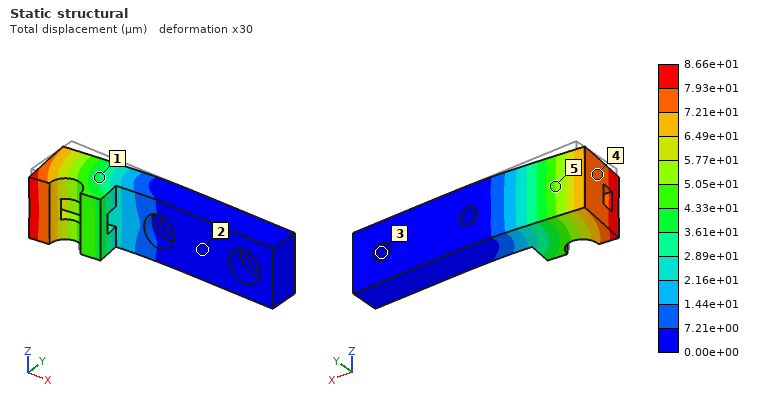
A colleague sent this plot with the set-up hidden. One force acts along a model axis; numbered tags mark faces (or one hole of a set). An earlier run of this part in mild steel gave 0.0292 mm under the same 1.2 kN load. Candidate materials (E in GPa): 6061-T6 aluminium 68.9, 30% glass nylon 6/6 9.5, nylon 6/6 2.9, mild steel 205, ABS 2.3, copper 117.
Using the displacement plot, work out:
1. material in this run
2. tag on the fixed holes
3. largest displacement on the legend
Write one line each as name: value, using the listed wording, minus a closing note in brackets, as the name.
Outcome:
material in this run: 6061-T6 aluminium
tag on the fixed holes: 3
largest displacement on the legend: 8.66e+01 µm
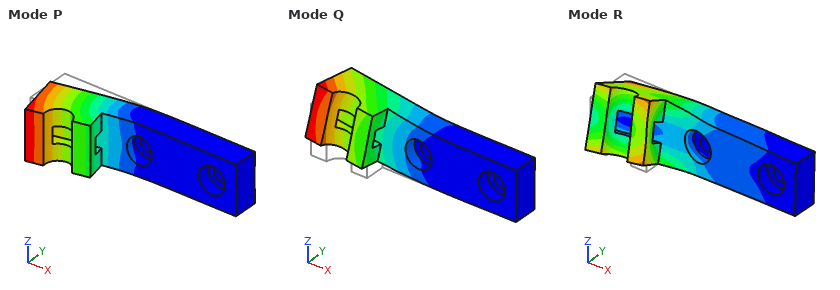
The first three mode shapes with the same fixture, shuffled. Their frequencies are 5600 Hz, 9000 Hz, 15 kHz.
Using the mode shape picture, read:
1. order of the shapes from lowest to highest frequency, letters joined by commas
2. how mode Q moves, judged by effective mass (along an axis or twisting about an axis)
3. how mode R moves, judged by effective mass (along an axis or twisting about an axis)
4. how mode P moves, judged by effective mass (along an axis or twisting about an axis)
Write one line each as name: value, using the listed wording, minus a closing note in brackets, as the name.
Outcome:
order of the shapes from lowest to highest frequency, letters joined by commas: P, Q, R
how mode Q moves, judged by effective mass: along Z
how mode R moves, judged by effective mass: twisting about X
how mode P moves, judged by effective mass: along Y
